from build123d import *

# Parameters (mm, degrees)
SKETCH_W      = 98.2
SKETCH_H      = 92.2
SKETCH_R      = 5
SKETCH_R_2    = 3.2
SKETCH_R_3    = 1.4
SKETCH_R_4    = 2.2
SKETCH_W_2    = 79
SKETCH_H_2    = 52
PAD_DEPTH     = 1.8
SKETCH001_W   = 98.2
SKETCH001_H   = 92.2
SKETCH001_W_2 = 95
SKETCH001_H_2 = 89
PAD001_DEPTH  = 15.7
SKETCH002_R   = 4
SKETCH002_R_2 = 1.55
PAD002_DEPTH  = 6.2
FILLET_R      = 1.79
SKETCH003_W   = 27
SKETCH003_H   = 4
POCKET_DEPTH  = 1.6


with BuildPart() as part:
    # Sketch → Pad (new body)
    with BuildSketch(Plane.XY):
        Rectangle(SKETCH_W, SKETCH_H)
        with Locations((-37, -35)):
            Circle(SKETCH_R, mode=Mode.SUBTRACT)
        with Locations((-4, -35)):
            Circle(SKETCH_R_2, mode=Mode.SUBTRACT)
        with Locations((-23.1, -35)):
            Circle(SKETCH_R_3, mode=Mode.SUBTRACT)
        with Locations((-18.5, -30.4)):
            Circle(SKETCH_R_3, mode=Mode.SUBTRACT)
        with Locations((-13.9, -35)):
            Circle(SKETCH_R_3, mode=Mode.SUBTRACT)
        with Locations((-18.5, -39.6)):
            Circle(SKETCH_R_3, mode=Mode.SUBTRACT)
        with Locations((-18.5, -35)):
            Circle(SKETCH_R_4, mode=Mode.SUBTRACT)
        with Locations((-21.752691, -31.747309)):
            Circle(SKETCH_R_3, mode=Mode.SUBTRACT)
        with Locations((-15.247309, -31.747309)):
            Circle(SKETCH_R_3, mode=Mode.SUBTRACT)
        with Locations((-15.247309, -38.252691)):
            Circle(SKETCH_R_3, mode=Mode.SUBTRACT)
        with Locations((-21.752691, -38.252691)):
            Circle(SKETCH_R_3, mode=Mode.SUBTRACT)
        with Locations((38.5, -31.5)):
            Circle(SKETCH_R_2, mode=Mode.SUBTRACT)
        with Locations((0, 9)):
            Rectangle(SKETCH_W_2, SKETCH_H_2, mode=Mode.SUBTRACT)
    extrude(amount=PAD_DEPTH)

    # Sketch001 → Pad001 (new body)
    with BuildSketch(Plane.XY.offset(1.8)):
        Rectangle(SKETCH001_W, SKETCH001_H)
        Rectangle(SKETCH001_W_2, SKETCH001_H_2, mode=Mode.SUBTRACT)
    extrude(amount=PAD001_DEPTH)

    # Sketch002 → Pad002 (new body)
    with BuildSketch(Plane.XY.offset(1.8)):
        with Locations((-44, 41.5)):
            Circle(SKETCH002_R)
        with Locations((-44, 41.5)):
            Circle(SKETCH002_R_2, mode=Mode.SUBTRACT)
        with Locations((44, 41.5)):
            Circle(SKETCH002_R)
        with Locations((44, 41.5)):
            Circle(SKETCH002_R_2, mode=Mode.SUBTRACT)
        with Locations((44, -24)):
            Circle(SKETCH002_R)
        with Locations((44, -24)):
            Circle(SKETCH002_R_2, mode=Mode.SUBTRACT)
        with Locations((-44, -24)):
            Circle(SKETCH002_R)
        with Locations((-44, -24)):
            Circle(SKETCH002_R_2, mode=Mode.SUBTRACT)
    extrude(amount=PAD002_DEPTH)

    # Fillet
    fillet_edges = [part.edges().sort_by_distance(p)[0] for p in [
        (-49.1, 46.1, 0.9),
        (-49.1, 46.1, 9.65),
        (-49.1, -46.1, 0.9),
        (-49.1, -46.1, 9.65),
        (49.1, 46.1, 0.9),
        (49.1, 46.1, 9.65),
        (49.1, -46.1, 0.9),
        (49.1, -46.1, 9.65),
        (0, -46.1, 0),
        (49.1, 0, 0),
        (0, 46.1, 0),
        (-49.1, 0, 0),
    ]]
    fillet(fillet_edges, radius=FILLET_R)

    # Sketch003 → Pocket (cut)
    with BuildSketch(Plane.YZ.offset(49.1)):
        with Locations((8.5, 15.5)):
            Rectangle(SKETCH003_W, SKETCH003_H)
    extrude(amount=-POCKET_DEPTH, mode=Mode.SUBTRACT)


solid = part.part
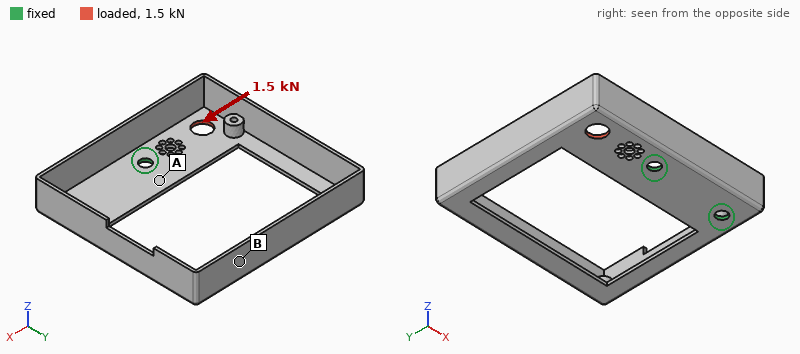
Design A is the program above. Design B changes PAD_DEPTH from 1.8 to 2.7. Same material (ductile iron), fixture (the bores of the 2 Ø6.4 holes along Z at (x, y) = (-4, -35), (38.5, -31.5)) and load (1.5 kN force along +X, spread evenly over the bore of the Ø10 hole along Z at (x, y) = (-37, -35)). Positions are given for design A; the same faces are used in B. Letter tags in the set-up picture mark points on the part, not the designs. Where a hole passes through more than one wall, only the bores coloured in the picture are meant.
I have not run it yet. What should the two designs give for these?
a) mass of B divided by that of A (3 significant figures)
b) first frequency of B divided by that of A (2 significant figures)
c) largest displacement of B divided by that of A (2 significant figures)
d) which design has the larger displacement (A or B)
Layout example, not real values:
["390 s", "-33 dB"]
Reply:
["1.19", "1.4", "0.73", "A"]
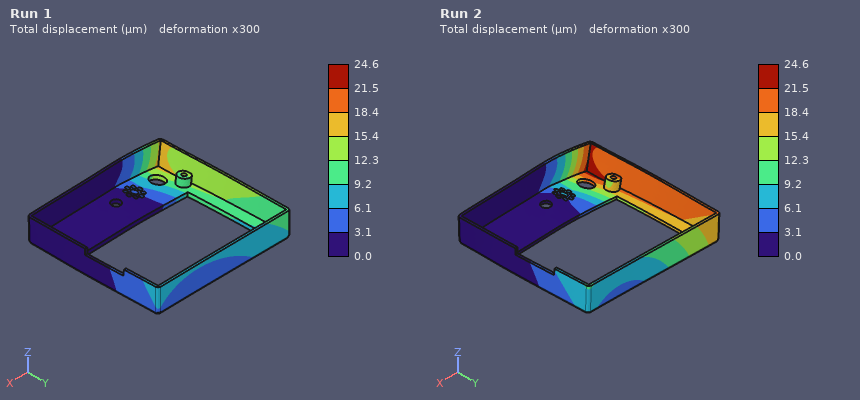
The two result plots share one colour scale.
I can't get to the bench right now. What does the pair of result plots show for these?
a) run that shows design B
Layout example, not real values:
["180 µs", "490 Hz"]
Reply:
["Run 1"]
